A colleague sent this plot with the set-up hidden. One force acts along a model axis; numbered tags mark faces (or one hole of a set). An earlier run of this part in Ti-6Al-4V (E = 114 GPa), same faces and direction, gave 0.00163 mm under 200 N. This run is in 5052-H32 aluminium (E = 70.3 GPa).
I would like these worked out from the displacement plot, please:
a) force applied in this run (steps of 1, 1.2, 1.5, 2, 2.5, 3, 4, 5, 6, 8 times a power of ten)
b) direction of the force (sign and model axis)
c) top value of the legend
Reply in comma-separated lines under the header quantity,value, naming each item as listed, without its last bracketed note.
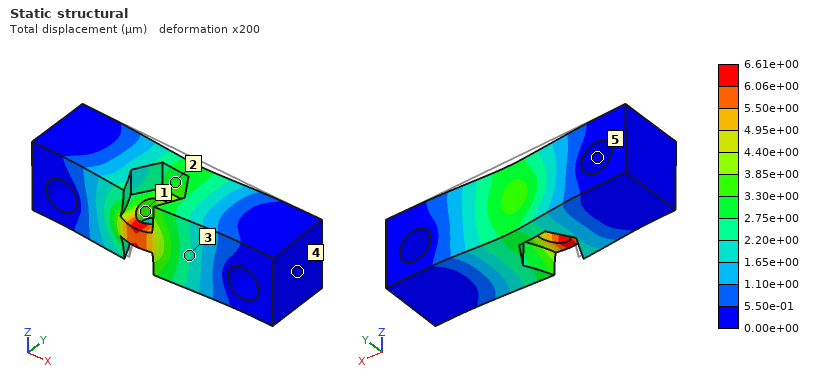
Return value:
quantity,value
force applied in this run,500 N
direction of the force,-Y
top value of the legend,6.61e+00 µm
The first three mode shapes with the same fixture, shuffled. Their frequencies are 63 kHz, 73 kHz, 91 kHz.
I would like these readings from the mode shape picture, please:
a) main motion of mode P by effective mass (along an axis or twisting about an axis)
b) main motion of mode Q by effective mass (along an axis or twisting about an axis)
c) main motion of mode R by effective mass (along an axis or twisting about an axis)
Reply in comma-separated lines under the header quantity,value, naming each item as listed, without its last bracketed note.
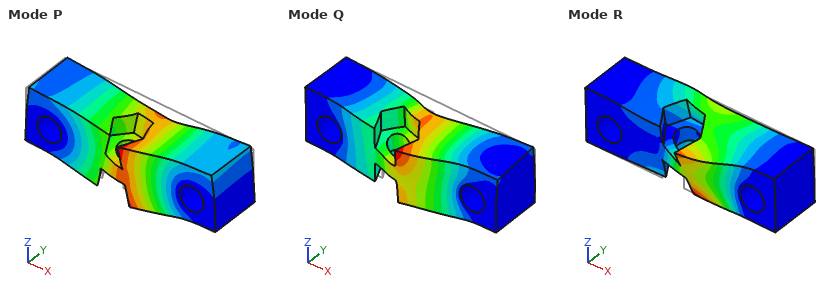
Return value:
quantity,value
main motion of mode P by effective mass,along Z
main motion of mode Q by effective mass,along Y
main motion of mode R by effective mass,twisting about X
